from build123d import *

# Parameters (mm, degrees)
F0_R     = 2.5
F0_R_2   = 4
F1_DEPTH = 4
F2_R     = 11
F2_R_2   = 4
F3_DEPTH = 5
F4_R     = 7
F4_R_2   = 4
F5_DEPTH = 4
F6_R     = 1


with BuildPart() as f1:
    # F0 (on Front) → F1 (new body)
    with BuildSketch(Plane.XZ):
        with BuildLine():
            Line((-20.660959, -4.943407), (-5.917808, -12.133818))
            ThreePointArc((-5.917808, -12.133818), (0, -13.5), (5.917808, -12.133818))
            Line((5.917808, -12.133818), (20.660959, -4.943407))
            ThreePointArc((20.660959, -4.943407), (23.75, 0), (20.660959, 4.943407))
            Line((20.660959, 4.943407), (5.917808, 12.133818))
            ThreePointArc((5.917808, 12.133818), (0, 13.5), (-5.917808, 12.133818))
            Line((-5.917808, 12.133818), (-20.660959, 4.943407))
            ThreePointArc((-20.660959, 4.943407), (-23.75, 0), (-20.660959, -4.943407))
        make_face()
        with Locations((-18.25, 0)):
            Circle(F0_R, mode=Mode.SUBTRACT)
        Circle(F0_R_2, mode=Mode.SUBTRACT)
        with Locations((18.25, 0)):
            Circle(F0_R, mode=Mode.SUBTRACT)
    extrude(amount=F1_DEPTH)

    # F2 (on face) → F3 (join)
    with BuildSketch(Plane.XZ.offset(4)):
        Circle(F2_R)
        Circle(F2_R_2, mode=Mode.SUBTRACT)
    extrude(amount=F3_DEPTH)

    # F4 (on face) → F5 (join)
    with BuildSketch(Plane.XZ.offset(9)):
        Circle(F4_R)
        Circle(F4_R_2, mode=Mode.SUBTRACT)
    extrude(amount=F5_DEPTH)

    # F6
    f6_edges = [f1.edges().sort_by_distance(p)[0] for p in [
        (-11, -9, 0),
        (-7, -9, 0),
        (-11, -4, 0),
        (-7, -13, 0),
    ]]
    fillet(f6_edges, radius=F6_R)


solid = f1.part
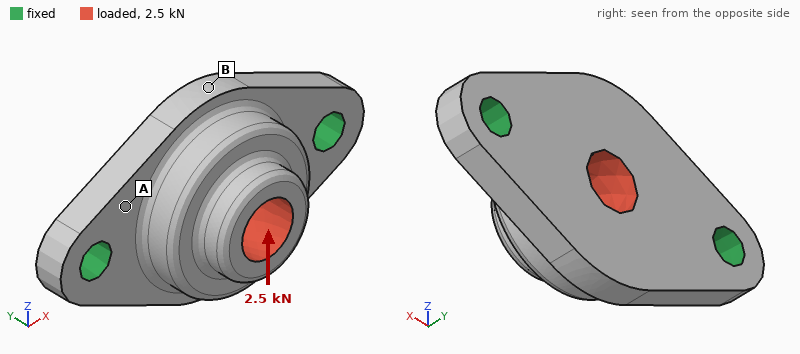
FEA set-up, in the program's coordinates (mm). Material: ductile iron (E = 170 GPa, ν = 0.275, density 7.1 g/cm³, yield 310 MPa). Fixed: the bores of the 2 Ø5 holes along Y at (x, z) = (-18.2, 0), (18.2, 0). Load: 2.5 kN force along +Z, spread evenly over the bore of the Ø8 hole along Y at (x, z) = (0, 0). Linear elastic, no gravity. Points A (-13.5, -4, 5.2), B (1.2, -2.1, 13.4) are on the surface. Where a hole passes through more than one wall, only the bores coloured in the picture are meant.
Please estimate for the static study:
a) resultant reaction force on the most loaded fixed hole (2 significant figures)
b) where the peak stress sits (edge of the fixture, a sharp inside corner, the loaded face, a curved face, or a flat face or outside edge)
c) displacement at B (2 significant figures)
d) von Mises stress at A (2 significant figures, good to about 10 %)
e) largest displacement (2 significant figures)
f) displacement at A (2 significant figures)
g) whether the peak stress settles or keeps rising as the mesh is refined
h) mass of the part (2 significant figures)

1.3 kN
edge of the fixture
24 µm
90 MPa
27 µm
6.7 µm
keeps rising
36 g
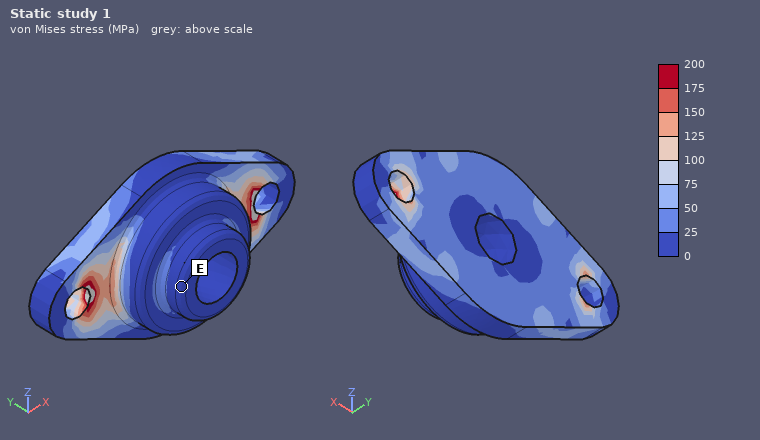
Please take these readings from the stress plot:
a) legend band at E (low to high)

0 to 25 MPa
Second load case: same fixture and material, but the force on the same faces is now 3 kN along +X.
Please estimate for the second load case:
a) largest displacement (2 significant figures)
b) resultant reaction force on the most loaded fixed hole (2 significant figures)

4.8 µm
1.6 kN
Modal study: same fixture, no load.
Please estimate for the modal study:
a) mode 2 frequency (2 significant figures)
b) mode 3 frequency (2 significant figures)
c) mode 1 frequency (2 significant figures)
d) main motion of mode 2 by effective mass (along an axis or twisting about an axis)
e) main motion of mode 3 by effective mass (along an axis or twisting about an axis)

15 kHz
26 kHz
9500 Hz
along Y
along Z
